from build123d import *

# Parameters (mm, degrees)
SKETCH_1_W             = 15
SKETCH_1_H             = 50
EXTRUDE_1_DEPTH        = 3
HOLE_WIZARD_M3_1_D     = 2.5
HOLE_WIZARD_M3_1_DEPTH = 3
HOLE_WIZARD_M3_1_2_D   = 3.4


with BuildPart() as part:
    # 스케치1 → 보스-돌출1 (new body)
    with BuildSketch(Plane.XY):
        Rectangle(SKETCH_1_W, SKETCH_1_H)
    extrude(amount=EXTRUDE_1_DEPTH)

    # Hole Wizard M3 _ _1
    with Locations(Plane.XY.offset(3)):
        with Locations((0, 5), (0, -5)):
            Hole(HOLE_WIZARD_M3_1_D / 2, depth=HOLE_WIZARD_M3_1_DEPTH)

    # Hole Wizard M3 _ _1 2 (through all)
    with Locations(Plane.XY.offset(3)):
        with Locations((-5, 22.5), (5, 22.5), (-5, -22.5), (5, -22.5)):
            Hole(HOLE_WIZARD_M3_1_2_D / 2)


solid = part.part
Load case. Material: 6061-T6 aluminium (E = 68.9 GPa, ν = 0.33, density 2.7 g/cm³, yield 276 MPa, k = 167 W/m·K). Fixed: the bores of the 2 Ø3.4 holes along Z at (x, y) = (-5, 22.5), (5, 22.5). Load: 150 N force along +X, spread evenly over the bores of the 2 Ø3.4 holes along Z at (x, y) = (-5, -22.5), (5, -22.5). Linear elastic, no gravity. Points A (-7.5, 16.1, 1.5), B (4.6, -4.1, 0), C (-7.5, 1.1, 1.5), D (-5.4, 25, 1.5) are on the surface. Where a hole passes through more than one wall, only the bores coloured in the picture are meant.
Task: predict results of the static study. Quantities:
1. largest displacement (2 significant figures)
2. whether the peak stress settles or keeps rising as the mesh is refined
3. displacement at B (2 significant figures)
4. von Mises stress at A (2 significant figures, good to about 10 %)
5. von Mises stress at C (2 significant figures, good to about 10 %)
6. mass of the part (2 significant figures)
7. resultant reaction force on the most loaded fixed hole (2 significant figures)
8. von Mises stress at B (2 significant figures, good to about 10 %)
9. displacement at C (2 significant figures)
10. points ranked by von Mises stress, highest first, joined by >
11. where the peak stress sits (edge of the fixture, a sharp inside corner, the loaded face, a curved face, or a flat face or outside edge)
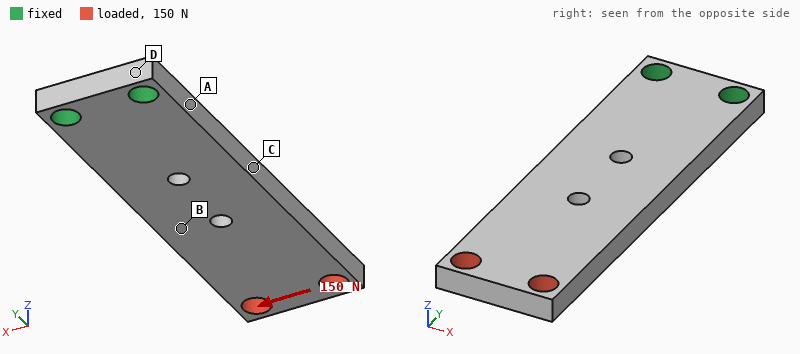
89 µm
keeps rising
35 µm
50 MPa
31 MPa
5.7 g
610 N
17 MPa
27 µm
A > C > B > D
edge of the fixture
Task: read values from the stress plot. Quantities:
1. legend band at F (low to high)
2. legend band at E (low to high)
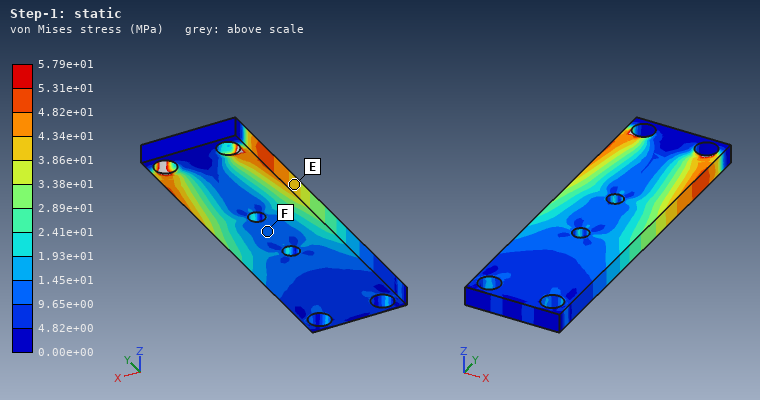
9.65e+00 to 1.45e+01 MPa
3.86e+01 to 4.34e+01 MPa
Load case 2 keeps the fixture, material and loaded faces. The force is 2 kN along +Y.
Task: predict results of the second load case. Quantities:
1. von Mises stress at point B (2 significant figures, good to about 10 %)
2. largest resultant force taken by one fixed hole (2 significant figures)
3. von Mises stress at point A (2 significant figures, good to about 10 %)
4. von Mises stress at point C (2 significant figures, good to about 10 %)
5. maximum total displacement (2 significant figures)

47 MPa
1.0 kN
46 MPa
50 MPa
41 µm
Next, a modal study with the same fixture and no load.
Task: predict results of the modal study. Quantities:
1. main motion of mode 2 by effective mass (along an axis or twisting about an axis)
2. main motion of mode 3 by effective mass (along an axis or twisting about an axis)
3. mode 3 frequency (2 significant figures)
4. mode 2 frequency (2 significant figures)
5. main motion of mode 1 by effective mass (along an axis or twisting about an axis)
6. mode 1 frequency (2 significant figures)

along X
twisting about Y
6800 Hz
5500 Hz
along Z
1200 Hz
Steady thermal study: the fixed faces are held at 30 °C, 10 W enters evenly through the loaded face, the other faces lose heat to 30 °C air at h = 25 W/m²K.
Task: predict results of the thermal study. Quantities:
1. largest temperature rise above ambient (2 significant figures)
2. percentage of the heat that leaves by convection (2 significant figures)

60 K
12 %
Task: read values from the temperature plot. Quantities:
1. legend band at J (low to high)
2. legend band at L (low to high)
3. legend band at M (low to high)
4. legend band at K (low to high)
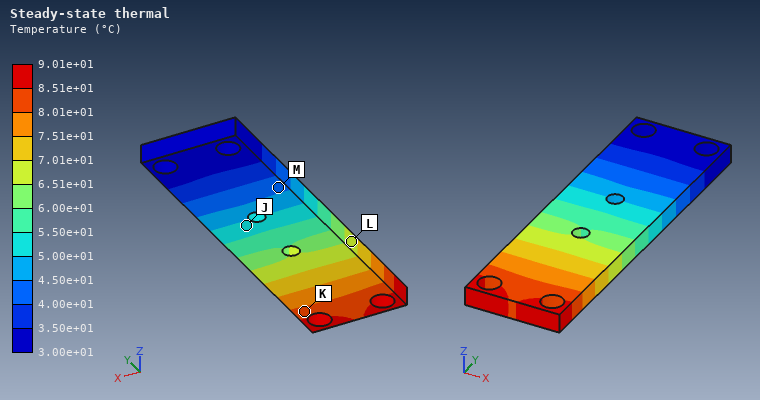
5.00e+01 to 5.50e+01 °C
6.51e+01 to 7.01e+01 °C
4.00e+01 to 4.50e+01 °C
8.01e+01 to 8.51e+01 °C
